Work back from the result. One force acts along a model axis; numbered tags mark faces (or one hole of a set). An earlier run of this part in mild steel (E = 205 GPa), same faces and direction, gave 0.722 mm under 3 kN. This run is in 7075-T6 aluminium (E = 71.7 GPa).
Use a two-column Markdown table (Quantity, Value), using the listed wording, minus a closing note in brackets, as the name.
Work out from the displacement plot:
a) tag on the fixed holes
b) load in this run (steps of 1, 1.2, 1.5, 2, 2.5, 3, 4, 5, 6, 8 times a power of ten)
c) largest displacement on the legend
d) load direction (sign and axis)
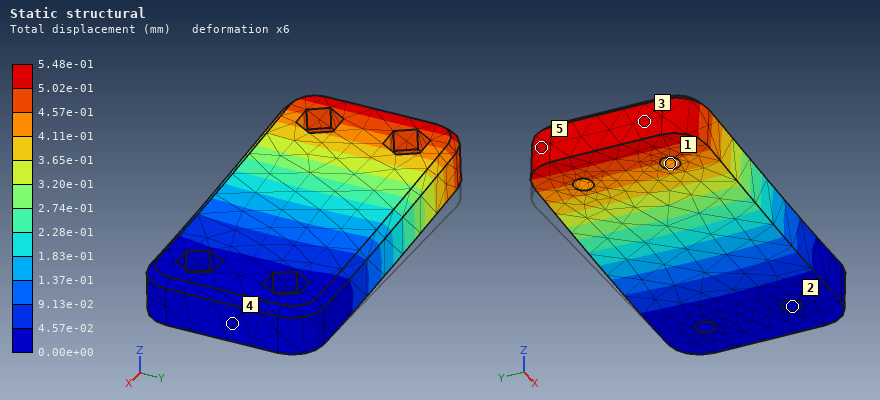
| Quantity | Value |
|---|---|
| tag on the fixed holes | 2 |
| load in this run | 800 N |
| largest displacement on the legend | 5.48e-01 mm |
| load direction | +Z |
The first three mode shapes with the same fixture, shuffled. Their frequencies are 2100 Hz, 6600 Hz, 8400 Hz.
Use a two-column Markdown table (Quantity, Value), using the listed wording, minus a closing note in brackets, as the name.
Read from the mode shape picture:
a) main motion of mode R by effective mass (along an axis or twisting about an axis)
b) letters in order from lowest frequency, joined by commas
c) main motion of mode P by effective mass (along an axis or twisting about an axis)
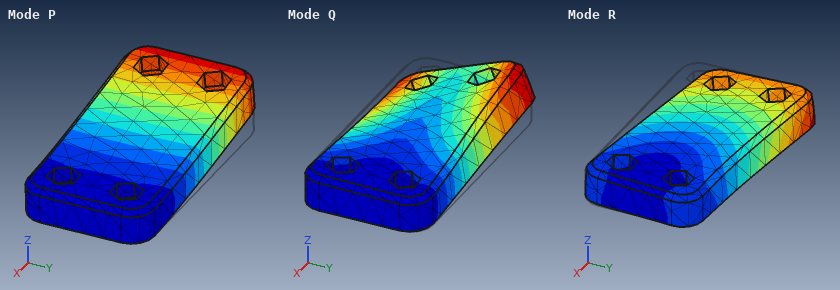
| Quantity | Value |
|---|---|
| main motion of mode R by effective mass | along Y |
| letters in order from lowest frequency, joined by commas | P, R, Q |
| main motion of mode P by effective mass | along Z |
